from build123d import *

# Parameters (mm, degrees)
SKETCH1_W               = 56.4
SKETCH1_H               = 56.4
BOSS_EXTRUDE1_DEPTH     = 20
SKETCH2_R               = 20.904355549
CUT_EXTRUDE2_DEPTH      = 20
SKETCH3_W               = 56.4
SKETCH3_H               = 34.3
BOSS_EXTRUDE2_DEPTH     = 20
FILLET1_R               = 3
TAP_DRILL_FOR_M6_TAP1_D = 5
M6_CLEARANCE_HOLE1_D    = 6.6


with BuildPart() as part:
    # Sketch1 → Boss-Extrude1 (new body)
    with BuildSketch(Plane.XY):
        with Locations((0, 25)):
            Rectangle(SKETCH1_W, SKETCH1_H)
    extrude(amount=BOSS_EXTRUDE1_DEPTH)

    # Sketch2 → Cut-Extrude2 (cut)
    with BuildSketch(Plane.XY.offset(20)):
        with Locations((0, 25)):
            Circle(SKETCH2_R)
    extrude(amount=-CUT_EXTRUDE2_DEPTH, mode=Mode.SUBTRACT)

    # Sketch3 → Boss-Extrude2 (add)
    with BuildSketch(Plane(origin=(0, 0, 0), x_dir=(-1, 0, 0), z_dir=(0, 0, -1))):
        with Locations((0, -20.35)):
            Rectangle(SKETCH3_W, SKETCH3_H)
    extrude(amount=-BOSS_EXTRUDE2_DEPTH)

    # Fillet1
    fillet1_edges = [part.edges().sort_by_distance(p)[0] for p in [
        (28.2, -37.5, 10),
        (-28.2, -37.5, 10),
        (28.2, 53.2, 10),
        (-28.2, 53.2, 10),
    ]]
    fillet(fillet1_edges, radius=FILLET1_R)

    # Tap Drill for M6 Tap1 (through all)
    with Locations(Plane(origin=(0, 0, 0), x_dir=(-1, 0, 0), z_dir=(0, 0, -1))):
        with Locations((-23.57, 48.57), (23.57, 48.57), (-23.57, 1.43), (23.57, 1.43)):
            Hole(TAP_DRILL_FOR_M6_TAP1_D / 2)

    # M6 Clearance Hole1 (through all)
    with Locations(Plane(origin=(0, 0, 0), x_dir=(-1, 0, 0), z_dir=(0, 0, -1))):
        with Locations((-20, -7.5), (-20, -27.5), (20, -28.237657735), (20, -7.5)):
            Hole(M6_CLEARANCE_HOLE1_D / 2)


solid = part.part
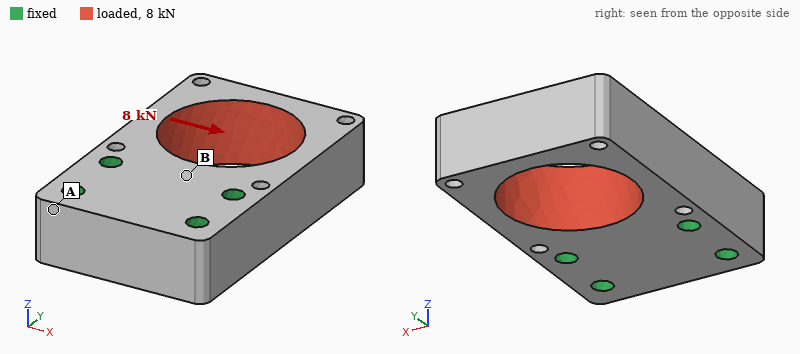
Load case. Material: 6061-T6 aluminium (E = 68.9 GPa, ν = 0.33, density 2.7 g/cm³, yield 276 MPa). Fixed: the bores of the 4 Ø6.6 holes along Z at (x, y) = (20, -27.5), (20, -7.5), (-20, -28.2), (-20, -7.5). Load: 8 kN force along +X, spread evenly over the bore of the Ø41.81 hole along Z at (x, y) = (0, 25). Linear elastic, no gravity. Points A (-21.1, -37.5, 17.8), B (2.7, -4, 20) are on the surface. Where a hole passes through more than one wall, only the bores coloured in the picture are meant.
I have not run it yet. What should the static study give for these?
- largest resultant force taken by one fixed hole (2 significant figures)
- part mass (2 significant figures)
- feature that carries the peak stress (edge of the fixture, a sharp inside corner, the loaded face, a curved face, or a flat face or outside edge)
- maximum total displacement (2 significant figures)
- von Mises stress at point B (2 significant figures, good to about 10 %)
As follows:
6.1 kN
190 g
a curved face
0.15 mm
27 MPa
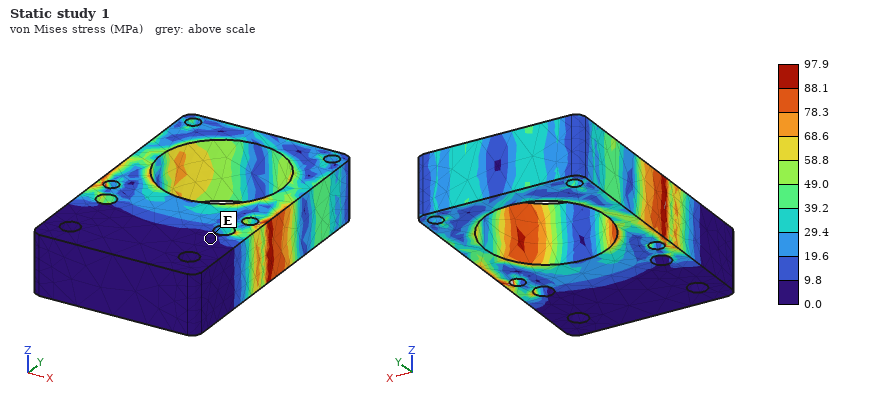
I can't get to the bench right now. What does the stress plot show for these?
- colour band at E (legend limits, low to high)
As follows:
0.0 to 9.8 MPa
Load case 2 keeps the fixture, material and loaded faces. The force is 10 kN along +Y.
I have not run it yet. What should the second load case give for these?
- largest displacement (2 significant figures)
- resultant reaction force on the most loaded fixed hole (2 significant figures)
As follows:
40 µm
4.5 kN
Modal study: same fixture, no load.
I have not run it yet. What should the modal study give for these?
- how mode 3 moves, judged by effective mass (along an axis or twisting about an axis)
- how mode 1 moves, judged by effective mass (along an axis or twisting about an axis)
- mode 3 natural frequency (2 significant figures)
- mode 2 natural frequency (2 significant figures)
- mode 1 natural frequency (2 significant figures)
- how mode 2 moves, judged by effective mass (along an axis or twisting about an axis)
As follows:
twisting about Y
along Z
6000 Hz
4100 Hz
3300 Hz
along X
